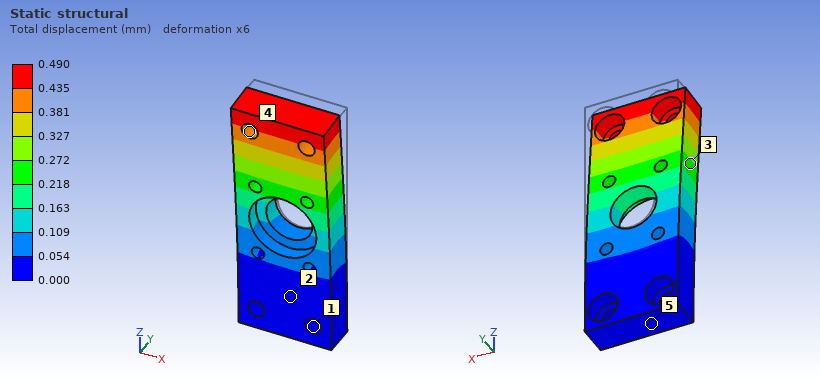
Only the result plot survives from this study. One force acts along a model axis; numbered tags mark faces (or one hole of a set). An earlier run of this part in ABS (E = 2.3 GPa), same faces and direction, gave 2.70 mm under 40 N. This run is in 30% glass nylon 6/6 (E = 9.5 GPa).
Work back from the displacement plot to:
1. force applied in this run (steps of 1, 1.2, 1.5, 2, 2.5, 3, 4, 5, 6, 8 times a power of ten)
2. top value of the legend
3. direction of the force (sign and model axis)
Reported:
30 N
0.490 mm
-Y
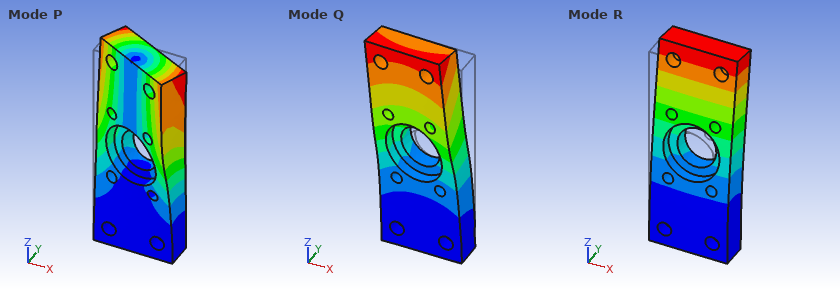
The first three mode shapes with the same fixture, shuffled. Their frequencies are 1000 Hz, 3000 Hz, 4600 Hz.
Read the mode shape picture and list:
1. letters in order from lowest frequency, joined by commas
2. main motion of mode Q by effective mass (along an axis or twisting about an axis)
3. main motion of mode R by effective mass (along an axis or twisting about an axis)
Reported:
R, Q, P
along X
along Y
